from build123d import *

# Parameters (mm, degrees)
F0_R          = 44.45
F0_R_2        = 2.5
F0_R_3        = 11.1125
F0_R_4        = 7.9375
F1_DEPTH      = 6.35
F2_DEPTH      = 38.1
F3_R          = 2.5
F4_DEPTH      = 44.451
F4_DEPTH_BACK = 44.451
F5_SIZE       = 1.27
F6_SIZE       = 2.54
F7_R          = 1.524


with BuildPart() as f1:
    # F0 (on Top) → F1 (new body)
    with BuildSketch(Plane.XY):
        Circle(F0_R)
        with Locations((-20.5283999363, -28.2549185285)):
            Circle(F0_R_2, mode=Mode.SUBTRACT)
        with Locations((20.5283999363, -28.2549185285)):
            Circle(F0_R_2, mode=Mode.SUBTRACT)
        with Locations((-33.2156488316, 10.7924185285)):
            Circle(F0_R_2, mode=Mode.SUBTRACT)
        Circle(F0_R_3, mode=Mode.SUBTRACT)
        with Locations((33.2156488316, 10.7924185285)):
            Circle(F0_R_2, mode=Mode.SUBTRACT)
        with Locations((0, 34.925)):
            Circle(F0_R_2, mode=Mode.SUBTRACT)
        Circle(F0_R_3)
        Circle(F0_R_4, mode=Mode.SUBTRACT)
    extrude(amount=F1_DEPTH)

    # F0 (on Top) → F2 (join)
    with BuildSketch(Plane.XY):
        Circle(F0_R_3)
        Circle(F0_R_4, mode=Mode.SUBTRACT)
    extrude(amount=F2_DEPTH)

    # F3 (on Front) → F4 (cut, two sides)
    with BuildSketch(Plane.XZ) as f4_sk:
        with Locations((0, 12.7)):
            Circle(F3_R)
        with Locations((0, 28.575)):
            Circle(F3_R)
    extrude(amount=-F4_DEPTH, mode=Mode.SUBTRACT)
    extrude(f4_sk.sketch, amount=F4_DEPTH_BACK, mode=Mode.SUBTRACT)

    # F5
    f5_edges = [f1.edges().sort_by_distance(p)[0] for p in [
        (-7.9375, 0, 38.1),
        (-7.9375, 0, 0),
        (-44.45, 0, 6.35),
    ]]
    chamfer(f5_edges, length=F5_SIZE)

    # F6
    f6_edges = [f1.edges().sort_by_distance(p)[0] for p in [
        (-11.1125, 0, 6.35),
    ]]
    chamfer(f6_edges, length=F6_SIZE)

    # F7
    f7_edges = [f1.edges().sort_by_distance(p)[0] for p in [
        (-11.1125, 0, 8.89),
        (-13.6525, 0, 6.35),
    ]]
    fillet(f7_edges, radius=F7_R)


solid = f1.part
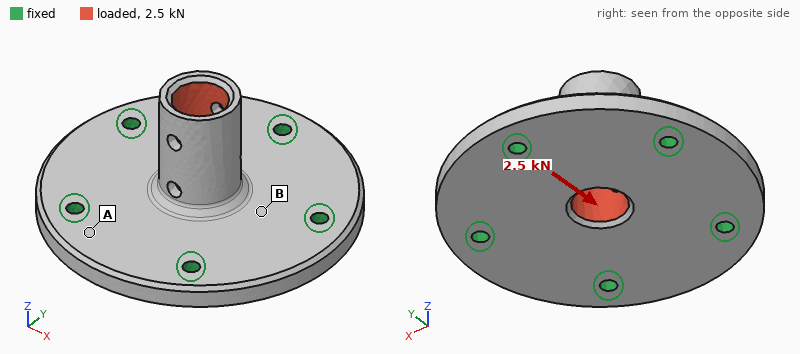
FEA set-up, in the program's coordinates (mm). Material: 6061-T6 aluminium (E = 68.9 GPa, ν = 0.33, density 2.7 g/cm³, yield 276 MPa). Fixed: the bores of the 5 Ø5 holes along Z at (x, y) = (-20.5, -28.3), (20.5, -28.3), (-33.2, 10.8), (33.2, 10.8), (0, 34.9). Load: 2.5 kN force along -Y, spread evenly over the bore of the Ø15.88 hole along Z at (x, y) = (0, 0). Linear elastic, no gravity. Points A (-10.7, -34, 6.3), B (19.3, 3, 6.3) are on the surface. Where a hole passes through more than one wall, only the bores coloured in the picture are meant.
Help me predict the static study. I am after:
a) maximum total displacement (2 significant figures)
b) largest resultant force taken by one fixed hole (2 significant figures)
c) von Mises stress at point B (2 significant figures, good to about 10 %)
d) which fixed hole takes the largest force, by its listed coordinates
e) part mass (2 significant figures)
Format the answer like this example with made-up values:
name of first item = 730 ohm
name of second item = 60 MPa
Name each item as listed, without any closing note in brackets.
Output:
maximum total displacement = 74 µm
largest resultant force taken by one fixed hole = 920 N
von Mises stress at point B = 17 MPa
which fixed hole takes the largest force, by its listed coordinates = (0, 34.9)
part mass = 120 g
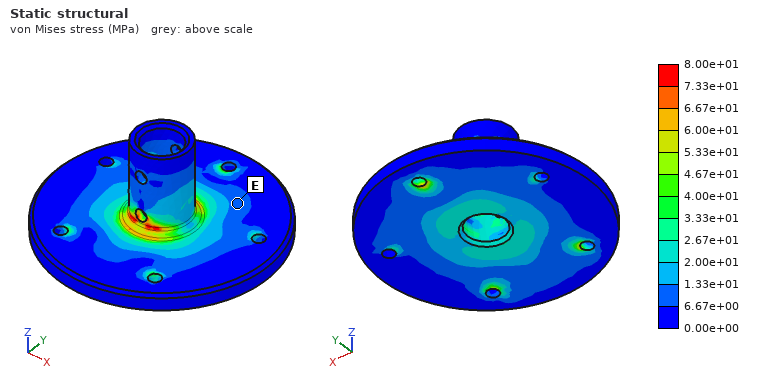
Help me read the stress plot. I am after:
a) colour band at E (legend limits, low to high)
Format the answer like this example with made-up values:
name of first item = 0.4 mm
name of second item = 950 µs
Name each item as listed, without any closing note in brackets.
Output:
colour band at E = 6.67e+00 to 1.33e+01 MPa
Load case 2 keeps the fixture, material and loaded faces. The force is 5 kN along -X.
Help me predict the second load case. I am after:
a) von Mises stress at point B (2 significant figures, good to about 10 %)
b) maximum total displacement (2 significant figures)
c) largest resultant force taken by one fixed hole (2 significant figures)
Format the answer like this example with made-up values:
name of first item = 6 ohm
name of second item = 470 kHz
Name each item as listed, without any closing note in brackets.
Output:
von Mises stress at point B = 39 MPa
maximum total displacement = 0.15 mm
largest resultant force taken by one fixed hole = 1.8 kN
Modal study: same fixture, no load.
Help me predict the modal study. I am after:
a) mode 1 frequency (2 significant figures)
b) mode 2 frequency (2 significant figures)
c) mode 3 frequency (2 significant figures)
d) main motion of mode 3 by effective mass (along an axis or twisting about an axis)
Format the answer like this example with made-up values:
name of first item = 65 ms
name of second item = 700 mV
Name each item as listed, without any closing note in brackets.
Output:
mode 1 frequency = 7600 Hz
mode 2 frequency = 7700 Hz
mode 3 frequency = 8400 Hz
main motion of mode 3 by effective mass = along Z
